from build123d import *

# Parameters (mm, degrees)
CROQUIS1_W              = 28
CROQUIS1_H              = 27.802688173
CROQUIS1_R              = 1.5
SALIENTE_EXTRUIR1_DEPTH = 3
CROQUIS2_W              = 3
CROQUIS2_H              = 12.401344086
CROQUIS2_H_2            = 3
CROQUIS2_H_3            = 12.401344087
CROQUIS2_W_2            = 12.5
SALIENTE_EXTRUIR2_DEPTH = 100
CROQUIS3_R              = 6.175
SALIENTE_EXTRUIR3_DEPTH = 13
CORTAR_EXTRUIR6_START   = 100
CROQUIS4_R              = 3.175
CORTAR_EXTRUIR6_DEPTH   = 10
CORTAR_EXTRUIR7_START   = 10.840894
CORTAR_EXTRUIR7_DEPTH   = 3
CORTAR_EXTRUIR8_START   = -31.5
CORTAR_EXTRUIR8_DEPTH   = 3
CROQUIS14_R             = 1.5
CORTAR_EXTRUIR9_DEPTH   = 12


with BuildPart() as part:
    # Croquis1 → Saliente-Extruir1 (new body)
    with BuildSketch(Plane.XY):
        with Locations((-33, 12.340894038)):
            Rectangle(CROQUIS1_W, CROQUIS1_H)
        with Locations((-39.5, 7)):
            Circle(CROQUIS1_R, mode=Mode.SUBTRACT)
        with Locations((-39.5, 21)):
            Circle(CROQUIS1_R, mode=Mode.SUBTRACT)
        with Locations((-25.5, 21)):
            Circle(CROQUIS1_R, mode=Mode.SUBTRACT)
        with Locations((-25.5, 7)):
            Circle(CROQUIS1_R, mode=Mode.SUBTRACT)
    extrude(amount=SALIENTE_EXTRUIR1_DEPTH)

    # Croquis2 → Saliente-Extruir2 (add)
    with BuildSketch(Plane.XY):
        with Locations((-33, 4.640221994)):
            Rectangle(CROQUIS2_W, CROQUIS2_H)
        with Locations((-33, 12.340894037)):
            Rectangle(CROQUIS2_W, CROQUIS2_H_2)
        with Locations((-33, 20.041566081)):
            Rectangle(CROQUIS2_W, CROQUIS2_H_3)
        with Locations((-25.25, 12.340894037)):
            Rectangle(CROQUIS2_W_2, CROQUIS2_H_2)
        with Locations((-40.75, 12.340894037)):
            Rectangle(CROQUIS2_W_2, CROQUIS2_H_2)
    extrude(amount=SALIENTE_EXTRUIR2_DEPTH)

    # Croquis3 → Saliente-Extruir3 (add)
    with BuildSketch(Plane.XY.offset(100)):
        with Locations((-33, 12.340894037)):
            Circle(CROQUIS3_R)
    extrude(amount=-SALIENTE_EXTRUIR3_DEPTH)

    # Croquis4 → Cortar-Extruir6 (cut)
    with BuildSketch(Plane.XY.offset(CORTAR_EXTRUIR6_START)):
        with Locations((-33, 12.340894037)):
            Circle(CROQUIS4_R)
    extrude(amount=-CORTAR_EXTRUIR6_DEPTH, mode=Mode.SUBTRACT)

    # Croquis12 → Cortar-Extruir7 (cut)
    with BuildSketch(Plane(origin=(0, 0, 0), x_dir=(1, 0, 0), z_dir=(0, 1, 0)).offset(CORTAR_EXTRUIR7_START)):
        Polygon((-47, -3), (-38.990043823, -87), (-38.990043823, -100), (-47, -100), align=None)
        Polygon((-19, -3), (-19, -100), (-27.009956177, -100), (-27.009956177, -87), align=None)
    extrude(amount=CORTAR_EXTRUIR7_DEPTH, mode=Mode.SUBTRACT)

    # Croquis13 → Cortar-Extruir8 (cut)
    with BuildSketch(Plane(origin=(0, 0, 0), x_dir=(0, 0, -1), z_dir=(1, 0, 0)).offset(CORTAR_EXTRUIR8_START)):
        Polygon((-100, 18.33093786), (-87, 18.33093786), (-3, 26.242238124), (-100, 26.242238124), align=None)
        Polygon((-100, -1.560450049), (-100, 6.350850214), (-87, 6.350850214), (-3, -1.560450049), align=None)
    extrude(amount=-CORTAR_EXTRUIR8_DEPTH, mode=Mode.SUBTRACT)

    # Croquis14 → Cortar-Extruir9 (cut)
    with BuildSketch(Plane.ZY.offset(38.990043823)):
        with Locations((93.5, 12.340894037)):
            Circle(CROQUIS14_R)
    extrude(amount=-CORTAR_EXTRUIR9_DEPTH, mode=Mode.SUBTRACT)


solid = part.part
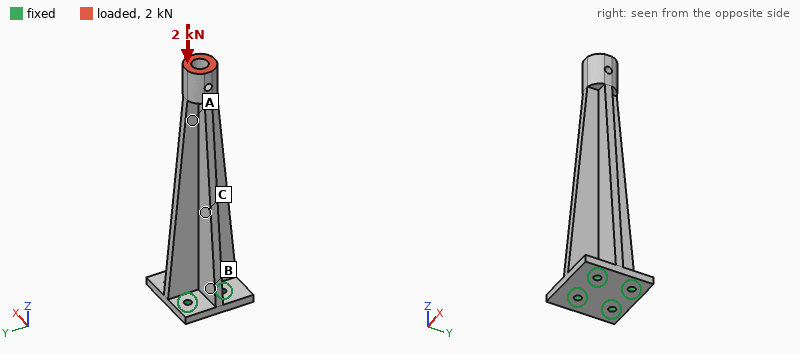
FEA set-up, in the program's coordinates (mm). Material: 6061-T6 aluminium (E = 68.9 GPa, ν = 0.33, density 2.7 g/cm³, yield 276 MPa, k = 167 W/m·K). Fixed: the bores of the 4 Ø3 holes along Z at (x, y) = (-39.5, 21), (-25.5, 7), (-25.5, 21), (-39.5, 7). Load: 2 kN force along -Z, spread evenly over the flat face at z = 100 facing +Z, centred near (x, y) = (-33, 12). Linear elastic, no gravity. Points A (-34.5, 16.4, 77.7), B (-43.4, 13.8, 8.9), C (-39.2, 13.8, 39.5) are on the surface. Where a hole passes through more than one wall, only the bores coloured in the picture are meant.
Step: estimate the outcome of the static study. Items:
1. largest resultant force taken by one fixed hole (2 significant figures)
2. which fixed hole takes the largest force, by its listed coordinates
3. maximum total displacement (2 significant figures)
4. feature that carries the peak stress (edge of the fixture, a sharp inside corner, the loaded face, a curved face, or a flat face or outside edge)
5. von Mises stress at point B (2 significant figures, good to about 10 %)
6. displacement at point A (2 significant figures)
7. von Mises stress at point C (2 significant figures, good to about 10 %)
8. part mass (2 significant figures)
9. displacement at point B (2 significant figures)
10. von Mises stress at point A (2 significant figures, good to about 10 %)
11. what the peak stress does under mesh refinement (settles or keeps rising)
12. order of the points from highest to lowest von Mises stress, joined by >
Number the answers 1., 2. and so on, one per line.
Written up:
1. 670 N
2. (-39.5, 7)
3. 35 µm
4. edge of the fixture
5. 12 MPa
6. 25 µm
7. 17 MPa
8. 34 g
9. 5.9 µm
10. 27 MPa
11. keeps rising
12. A > C > B
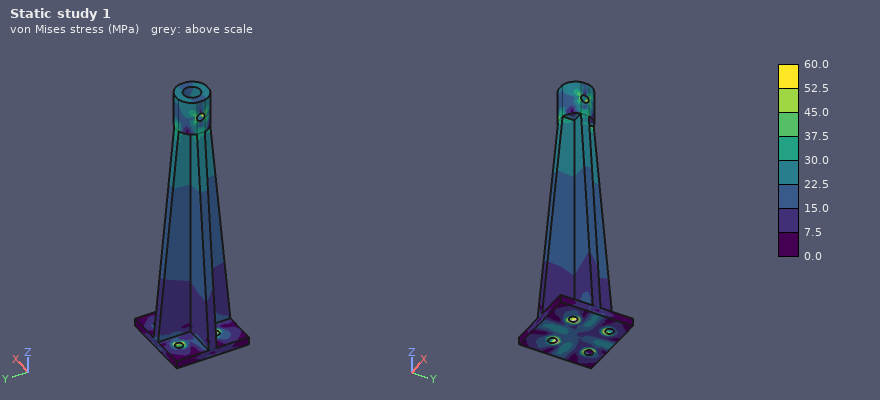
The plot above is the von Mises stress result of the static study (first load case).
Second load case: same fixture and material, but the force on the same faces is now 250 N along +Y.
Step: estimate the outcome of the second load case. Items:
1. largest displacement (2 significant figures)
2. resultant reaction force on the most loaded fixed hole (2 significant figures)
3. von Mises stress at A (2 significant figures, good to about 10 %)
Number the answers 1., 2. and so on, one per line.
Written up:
1. 0.60 mm
2. 850 N
3. 34 MPa
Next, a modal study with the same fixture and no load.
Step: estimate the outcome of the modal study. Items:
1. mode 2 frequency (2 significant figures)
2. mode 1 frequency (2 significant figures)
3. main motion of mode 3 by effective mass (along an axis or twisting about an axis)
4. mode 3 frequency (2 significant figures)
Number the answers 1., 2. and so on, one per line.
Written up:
1. 1500 Hz
2. 1400 Hz
3. twisting about Z
4. 3500 Hz
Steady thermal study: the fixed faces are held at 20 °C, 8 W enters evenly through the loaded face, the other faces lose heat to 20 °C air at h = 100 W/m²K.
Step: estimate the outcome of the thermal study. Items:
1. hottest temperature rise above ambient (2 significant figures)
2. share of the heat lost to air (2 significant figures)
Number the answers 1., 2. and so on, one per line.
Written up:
1. 26 K
2. 72 %
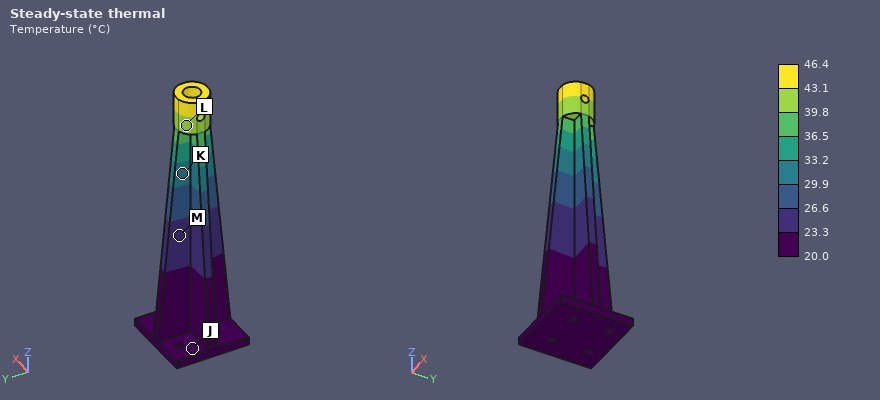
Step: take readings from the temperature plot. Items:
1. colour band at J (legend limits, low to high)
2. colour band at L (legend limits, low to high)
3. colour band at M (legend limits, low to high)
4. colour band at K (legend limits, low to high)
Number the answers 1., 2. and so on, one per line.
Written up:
1. 20.0 to 23.3 °C
2. 39.8 to 43.1 °C
3. 23.3 to 26.6 °C
4. 29.9 to 33.2 °C
